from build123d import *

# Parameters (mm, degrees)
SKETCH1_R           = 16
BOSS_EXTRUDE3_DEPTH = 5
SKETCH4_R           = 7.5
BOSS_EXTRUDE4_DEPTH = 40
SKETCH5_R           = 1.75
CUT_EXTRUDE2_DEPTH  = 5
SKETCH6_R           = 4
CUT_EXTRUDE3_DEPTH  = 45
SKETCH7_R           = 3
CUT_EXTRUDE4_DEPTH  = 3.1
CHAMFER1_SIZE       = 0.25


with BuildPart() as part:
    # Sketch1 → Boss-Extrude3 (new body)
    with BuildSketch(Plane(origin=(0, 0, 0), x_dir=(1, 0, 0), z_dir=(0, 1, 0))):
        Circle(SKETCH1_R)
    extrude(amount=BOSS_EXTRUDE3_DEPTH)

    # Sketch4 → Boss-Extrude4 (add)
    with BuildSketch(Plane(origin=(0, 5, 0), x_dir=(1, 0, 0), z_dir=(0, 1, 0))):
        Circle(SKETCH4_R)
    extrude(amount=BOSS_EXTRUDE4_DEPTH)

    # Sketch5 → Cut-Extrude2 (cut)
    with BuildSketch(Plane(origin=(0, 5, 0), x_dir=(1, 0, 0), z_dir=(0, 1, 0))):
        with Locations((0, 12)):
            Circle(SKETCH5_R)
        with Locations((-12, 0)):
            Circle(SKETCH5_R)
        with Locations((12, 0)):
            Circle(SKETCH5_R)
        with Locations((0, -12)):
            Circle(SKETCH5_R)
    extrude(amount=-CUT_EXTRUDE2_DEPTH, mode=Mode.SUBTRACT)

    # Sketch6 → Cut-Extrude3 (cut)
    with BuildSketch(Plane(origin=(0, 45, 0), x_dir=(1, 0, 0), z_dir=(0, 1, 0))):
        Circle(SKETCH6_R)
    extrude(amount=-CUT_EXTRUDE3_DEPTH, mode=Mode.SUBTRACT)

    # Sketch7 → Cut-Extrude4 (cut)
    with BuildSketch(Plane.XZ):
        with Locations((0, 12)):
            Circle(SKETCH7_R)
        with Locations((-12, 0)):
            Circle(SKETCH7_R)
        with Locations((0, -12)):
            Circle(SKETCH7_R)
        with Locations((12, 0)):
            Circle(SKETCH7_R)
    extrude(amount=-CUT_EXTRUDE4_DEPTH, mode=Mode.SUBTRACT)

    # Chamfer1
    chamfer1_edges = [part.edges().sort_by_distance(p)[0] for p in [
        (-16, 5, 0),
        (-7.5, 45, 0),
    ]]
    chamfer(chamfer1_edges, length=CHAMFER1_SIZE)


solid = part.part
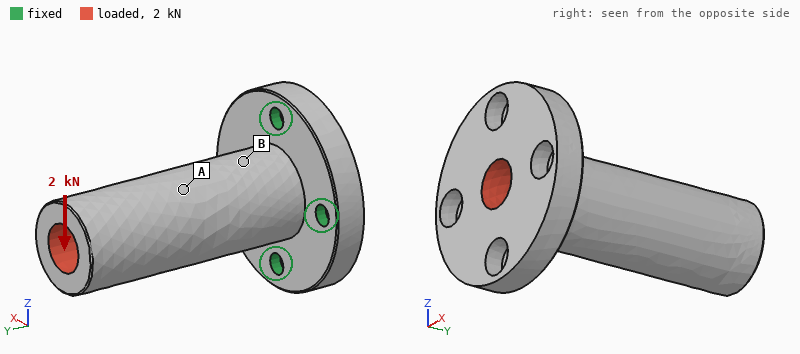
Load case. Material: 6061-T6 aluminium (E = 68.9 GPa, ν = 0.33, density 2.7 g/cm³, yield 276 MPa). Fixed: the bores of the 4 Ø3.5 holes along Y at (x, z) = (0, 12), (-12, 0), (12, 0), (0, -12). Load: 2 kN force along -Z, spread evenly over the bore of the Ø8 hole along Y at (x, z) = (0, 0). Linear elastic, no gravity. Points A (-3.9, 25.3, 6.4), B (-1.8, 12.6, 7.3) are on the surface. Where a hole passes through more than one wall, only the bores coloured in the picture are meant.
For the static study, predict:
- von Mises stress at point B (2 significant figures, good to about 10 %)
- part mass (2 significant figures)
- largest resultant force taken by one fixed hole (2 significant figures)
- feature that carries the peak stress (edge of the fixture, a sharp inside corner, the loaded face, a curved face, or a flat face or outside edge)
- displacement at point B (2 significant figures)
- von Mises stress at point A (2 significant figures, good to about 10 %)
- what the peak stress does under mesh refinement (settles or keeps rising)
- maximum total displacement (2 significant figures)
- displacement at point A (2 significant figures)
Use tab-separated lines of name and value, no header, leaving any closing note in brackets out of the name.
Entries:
von Mises stress at point B	71 MPa
part mass	23 g
largest resultant force taken by one fixed hole	1.6 kN
feature that carries the peak stress	edge of the fixture
displacement at point B	0.043 mm
von Mises stress at point A	26 MPa
what the peak stress does under mesh refinement	keeps rising
maximum total displacement	0.21 mm
displacement at point A	0.10 mm
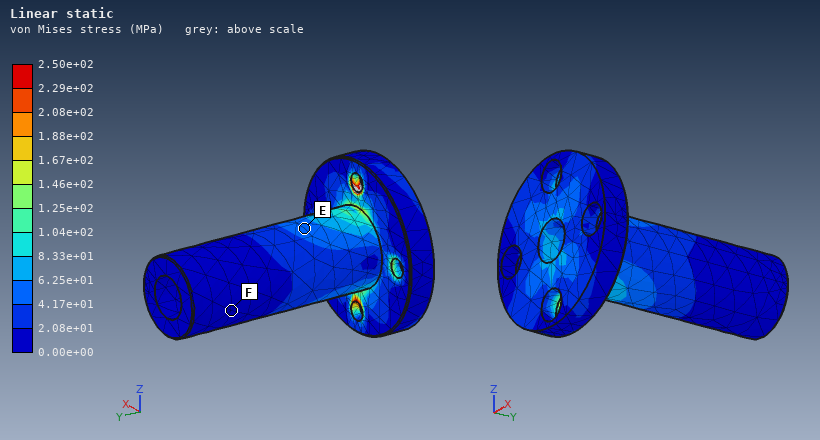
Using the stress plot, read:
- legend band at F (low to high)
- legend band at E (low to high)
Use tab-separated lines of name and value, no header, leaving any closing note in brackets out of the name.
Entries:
legend band at F	0.00e+00 to 2.08e+01 MPa
legend band at E	4.17e+01 to 6.25e+01 MPa
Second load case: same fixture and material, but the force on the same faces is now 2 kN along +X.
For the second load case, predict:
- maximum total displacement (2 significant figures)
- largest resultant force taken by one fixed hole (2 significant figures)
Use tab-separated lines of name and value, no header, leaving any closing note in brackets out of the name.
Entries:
maximum total displacement	0.21 mm
largest resultant force taken by one fixed hole	1.6 kN
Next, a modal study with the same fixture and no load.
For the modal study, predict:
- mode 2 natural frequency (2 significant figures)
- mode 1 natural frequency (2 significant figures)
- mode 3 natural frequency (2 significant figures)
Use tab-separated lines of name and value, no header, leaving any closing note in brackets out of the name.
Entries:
mode 2 natural frequency	4900 Hz
mode 1 natural frequency	4900 Hz
mode 3 natural frequency	18 kHz
